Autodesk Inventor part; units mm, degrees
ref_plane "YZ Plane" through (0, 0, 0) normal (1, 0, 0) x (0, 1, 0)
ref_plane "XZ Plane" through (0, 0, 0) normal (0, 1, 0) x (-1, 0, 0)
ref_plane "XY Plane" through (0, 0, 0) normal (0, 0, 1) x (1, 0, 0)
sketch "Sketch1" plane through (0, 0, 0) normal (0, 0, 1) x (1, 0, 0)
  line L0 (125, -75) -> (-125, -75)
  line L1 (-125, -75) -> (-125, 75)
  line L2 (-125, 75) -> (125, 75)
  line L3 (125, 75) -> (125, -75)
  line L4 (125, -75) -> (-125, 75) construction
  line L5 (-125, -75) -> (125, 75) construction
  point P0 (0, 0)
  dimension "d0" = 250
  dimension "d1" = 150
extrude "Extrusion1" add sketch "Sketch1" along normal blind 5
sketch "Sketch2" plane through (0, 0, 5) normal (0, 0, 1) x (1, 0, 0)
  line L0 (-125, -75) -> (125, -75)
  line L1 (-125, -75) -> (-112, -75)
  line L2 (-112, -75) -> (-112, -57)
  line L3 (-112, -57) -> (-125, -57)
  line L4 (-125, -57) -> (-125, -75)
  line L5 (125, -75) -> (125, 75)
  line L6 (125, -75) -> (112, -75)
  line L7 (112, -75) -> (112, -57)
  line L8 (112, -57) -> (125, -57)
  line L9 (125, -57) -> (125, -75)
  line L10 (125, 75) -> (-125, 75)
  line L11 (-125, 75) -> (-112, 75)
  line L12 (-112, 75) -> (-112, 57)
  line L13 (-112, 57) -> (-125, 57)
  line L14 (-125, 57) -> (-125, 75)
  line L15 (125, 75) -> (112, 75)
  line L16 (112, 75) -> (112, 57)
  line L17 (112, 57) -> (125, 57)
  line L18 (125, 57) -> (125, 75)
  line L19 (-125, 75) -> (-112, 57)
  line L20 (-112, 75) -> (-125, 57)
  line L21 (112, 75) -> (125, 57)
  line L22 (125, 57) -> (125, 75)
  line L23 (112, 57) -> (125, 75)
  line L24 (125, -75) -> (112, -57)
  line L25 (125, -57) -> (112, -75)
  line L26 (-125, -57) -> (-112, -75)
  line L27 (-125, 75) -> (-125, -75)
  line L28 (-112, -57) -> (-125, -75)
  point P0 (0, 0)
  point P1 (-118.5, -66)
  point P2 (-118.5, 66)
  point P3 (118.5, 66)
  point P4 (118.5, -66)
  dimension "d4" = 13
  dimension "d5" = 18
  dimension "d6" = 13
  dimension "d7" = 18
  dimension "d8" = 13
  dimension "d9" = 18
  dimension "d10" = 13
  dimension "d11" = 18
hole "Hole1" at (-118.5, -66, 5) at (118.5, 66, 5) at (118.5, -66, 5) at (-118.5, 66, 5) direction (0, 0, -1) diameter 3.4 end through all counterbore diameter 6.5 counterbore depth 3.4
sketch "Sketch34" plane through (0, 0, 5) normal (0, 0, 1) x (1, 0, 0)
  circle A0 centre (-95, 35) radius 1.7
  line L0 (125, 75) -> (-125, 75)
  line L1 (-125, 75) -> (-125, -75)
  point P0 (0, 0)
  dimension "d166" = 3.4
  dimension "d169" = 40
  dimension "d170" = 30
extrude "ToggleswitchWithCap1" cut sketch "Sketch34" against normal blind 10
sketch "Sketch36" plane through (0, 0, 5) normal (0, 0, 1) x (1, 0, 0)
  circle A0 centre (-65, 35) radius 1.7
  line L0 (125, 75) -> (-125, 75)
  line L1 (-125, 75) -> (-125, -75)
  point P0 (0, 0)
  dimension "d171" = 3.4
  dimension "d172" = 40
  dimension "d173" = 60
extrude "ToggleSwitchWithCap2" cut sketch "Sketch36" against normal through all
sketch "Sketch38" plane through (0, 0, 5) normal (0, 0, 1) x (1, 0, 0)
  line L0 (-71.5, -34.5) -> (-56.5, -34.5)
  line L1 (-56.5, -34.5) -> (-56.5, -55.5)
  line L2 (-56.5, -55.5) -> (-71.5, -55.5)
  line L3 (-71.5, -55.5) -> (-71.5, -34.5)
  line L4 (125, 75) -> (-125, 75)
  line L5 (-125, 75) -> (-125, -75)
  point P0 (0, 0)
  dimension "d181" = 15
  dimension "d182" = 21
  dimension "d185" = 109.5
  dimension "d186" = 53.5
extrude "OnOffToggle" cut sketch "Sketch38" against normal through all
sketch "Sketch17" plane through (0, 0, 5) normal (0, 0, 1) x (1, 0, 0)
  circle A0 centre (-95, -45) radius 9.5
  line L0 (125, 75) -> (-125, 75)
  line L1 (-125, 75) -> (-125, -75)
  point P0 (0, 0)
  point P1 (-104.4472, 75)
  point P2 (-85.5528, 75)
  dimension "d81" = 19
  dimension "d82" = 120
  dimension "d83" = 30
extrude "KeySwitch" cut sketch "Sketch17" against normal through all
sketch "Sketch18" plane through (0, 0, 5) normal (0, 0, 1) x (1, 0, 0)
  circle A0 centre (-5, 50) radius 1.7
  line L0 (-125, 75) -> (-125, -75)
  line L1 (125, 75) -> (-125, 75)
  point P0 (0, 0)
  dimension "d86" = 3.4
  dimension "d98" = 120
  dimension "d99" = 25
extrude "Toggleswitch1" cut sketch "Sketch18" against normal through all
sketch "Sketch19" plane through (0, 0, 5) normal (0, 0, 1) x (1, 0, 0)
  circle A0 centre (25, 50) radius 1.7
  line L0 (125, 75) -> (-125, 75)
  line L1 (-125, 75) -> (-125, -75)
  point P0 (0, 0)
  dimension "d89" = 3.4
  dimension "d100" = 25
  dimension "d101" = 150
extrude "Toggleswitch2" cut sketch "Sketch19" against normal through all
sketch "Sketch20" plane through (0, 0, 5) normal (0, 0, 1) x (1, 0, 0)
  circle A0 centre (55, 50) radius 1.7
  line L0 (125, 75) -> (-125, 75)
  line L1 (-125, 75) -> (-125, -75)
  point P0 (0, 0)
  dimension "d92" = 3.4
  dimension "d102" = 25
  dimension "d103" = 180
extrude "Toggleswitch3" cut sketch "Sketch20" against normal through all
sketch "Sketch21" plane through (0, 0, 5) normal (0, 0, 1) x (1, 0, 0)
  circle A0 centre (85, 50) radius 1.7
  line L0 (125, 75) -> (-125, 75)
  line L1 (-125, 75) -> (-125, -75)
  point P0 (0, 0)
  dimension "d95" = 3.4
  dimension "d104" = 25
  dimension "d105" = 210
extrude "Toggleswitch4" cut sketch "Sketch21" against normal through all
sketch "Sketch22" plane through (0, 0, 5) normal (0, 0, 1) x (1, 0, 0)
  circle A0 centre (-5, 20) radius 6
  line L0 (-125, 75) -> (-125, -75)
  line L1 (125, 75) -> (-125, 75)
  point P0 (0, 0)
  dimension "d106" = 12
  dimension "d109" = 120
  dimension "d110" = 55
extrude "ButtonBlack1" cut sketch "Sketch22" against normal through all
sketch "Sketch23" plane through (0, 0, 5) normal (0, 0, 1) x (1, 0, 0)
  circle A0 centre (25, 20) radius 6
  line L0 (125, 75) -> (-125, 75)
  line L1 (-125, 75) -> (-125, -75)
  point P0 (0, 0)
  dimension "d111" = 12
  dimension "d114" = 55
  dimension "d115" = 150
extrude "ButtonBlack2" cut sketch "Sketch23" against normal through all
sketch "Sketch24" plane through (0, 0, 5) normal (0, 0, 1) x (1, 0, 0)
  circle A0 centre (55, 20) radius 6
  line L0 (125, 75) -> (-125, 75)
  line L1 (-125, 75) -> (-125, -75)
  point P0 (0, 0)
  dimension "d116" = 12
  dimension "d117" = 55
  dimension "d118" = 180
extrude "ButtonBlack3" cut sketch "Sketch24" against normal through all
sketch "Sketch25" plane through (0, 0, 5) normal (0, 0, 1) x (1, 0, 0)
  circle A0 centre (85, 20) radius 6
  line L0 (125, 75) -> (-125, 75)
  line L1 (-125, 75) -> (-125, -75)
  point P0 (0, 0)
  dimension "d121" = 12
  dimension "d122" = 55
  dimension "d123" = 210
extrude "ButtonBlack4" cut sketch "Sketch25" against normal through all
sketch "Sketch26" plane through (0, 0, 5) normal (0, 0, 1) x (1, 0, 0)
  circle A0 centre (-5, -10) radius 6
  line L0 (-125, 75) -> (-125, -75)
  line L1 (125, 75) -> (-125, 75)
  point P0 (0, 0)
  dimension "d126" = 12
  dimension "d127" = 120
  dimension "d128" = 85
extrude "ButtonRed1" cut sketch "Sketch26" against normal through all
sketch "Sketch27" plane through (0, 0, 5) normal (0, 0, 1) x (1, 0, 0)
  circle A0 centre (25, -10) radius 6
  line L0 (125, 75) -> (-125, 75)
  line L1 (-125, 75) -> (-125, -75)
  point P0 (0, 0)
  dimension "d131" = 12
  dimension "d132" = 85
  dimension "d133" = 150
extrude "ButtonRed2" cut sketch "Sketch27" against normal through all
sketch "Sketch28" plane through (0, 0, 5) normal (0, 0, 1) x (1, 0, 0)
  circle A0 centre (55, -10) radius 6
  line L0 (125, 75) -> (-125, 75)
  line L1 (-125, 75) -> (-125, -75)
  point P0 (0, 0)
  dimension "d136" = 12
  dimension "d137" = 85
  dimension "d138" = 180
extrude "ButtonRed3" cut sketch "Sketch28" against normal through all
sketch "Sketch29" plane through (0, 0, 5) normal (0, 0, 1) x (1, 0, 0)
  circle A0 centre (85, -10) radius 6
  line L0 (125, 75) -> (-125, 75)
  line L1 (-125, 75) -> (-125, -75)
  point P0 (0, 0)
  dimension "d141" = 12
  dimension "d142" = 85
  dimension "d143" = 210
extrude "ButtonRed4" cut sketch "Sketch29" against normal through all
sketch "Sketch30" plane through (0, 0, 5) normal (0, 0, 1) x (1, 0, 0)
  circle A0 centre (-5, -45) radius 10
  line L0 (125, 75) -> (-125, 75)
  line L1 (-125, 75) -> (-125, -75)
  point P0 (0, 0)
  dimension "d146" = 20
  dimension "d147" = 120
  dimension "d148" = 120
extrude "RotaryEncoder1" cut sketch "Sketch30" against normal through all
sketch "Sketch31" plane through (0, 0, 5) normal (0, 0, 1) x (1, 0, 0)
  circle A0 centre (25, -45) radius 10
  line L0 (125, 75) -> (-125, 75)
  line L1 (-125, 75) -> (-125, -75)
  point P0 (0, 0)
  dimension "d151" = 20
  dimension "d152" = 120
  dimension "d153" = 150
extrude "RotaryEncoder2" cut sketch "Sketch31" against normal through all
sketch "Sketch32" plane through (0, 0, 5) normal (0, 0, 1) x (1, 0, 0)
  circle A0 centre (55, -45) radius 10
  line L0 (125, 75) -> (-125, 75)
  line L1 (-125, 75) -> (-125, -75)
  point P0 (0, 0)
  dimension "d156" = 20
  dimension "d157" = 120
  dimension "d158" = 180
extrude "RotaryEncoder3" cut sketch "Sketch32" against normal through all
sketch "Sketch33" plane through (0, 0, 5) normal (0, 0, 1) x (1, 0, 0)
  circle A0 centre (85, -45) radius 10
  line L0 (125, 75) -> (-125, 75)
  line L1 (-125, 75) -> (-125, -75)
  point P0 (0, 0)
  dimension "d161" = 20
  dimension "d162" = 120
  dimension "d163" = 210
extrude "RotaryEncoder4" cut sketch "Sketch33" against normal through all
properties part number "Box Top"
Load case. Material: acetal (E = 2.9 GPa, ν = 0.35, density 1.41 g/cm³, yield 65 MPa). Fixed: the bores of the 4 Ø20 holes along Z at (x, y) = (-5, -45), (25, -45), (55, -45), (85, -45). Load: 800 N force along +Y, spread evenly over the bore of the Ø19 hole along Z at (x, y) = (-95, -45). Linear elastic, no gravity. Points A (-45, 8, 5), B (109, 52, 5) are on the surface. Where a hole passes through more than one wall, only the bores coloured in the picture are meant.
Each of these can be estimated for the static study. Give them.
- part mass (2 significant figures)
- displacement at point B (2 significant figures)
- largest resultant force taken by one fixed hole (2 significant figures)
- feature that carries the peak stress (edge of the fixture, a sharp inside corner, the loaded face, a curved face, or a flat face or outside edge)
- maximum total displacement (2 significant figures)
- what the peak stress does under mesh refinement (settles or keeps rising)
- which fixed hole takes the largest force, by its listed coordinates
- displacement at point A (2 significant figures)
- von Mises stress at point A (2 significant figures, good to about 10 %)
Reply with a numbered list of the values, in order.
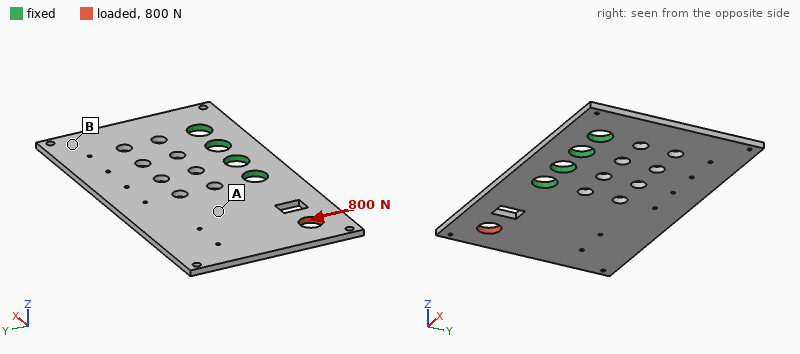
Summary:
1. 240 g
2. 0.18 mm
3. 1.4 kN
4. edge of the fixture
5. 0.55 mm
6. keeps rising
7. (-5, -45)
8. 0.21 mm
9. 2.6 MPa
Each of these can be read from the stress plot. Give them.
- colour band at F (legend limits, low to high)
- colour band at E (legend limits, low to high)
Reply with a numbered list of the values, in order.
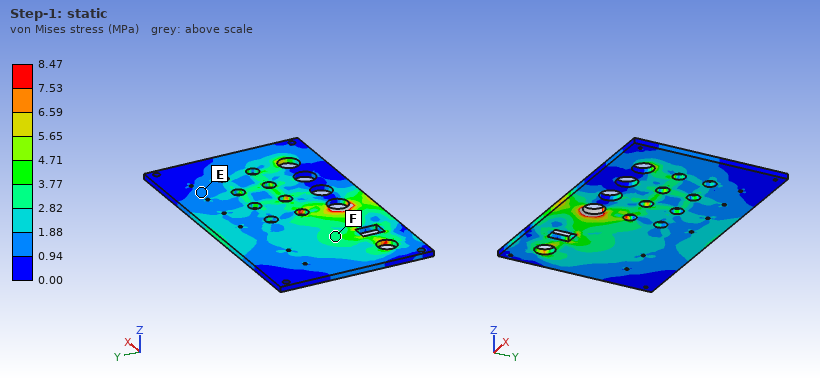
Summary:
1. 2.82 to 3.77 MPa
2. 0.94 to 1.88 MPa
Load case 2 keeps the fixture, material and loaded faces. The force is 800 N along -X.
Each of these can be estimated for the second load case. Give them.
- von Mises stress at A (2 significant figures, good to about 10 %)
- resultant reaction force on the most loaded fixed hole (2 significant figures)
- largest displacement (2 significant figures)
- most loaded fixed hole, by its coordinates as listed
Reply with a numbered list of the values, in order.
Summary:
1. 0.61 MPa
2. 620 N
3. 0.13 mm
4. (-5, -45)
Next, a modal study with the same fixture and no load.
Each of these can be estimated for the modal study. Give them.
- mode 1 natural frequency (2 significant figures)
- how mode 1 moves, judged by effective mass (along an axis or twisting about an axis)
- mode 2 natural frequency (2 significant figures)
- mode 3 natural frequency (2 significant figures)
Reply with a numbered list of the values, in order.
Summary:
1. 60 Hz
2. along Z
3. 93 Hz
4. 140 Hz
